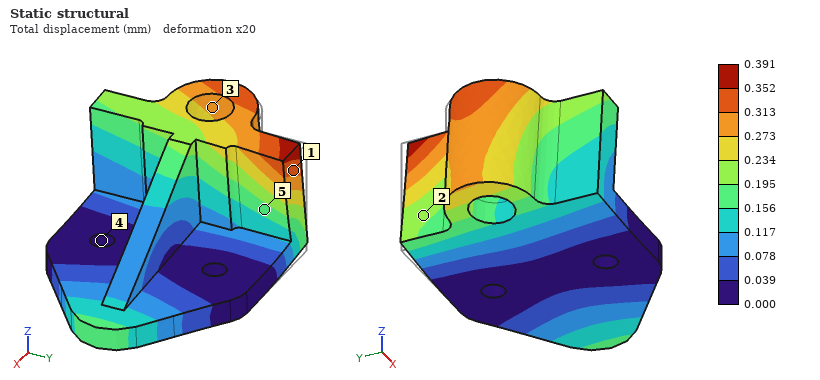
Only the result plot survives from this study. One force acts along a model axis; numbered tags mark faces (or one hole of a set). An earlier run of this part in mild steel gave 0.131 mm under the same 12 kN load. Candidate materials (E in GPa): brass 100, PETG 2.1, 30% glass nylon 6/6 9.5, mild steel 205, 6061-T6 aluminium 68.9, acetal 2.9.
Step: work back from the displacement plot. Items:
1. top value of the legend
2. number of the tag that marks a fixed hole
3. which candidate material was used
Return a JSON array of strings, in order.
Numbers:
["0.391 mm", "4", "6061-T6 aluminium"]
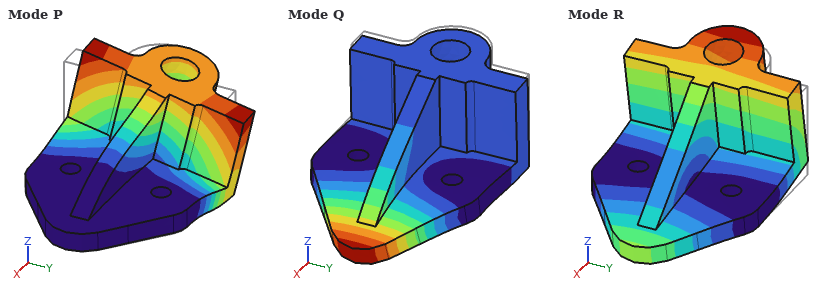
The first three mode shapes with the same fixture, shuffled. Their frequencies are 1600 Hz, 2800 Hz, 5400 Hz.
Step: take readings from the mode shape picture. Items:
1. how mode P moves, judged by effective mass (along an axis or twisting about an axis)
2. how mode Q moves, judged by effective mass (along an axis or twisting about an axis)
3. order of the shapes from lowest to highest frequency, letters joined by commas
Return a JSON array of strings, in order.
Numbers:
["along Y", "along Z", "R, P, Q"]
